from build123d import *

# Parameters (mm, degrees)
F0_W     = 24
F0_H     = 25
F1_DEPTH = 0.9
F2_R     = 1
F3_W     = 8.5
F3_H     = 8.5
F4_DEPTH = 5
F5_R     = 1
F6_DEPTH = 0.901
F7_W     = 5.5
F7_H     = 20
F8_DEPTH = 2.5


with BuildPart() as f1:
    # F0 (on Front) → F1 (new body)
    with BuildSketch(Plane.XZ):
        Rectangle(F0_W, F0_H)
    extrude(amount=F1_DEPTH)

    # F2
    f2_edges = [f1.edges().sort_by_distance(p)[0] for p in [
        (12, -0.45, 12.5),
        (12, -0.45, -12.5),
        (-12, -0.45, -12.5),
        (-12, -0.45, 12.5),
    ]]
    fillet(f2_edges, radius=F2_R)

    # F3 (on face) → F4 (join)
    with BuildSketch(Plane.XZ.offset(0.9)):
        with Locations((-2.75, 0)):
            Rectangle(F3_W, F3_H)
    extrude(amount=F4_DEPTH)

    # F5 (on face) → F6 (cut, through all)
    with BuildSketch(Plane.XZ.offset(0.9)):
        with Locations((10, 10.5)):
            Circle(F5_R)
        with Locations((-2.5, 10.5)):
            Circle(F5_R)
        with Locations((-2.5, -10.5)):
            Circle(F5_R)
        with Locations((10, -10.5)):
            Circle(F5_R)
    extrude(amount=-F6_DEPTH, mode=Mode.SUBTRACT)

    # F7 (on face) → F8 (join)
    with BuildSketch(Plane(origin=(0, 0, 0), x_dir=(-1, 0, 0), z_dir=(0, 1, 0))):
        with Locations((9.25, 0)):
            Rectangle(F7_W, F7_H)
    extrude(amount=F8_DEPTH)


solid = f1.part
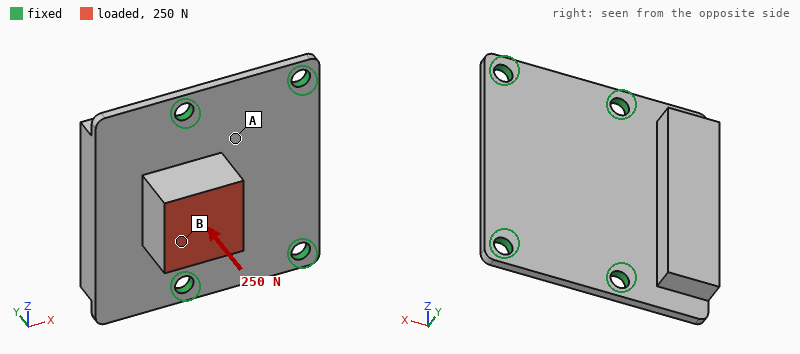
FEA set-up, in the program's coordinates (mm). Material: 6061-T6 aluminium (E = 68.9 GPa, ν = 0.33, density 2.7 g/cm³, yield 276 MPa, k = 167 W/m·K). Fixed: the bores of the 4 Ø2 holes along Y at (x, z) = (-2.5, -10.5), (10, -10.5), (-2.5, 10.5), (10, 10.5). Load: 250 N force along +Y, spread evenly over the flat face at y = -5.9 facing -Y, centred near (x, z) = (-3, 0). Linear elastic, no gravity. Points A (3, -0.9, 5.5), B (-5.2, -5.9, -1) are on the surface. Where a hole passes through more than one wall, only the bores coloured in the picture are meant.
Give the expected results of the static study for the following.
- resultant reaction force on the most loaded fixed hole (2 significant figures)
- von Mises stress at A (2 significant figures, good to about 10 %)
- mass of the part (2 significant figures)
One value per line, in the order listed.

120 N
39 MPa
3.1 g
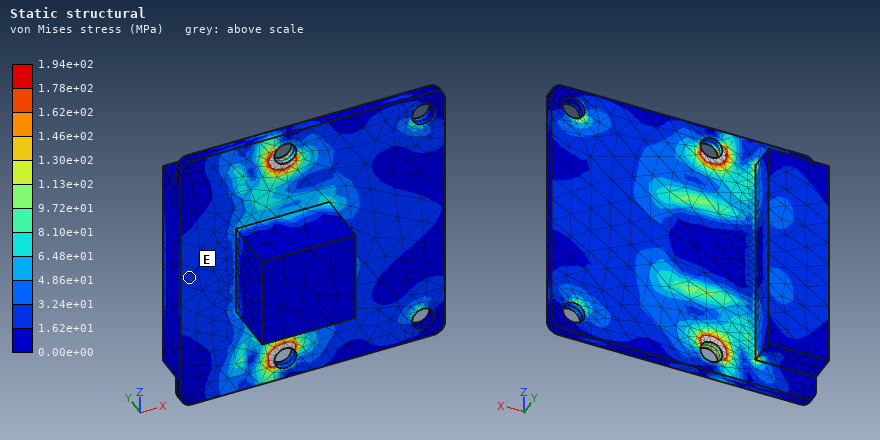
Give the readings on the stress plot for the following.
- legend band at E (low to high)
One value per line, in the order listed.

1.62e+01 to 3.24e+01 MPa
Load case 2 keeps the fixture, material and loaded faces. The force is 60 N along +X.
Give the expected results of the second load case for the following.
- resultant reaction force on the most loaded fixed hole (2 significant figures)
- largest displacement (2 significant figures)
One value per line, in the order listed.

24 N
32 µm
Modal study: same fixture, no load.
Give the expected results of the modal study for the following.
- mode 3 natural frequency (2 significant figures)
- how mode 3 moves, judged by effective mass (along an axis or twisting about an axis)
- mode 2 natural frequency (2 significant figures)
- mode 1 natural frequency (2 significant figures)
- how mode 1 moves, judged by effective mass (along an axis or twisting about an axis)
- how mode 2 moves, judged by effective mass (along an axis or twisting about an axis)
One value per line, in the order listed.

15 kHz
twisting about X
9800 Hz
5200 Hz
along Y
along Y
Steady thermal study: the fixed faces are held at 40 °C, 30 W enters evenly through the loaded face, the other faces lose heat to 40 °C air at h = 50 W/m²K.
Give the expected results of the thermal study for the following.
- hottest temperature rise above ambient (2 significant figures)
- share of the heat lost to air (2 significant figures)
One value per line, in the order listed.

58 K
6.6 %
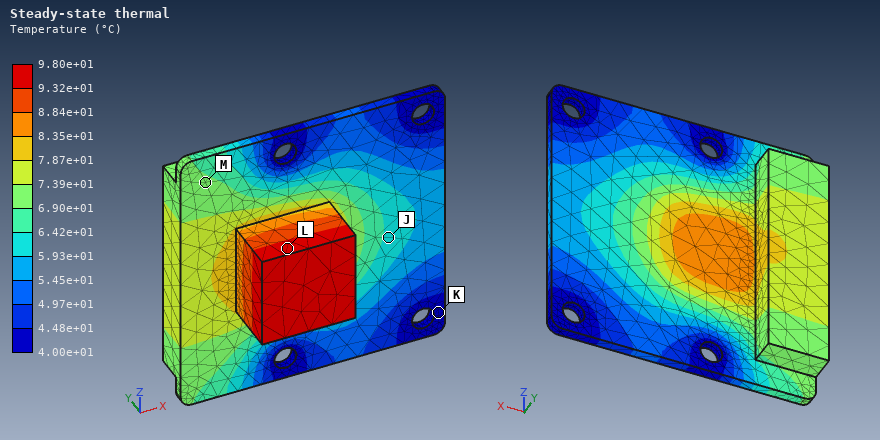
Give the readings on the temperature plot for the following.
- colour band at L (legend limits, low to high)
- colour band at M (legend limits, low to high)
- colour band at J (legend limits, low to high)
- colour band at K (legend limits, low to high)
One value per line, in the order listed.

9.32e+01 to 9.80e+01 °C
6.90e+01 to 7.39e+01 °C
5.93e+01 to 6.42e+01 °C
4.00e+01 to 4.48e+01 °C
